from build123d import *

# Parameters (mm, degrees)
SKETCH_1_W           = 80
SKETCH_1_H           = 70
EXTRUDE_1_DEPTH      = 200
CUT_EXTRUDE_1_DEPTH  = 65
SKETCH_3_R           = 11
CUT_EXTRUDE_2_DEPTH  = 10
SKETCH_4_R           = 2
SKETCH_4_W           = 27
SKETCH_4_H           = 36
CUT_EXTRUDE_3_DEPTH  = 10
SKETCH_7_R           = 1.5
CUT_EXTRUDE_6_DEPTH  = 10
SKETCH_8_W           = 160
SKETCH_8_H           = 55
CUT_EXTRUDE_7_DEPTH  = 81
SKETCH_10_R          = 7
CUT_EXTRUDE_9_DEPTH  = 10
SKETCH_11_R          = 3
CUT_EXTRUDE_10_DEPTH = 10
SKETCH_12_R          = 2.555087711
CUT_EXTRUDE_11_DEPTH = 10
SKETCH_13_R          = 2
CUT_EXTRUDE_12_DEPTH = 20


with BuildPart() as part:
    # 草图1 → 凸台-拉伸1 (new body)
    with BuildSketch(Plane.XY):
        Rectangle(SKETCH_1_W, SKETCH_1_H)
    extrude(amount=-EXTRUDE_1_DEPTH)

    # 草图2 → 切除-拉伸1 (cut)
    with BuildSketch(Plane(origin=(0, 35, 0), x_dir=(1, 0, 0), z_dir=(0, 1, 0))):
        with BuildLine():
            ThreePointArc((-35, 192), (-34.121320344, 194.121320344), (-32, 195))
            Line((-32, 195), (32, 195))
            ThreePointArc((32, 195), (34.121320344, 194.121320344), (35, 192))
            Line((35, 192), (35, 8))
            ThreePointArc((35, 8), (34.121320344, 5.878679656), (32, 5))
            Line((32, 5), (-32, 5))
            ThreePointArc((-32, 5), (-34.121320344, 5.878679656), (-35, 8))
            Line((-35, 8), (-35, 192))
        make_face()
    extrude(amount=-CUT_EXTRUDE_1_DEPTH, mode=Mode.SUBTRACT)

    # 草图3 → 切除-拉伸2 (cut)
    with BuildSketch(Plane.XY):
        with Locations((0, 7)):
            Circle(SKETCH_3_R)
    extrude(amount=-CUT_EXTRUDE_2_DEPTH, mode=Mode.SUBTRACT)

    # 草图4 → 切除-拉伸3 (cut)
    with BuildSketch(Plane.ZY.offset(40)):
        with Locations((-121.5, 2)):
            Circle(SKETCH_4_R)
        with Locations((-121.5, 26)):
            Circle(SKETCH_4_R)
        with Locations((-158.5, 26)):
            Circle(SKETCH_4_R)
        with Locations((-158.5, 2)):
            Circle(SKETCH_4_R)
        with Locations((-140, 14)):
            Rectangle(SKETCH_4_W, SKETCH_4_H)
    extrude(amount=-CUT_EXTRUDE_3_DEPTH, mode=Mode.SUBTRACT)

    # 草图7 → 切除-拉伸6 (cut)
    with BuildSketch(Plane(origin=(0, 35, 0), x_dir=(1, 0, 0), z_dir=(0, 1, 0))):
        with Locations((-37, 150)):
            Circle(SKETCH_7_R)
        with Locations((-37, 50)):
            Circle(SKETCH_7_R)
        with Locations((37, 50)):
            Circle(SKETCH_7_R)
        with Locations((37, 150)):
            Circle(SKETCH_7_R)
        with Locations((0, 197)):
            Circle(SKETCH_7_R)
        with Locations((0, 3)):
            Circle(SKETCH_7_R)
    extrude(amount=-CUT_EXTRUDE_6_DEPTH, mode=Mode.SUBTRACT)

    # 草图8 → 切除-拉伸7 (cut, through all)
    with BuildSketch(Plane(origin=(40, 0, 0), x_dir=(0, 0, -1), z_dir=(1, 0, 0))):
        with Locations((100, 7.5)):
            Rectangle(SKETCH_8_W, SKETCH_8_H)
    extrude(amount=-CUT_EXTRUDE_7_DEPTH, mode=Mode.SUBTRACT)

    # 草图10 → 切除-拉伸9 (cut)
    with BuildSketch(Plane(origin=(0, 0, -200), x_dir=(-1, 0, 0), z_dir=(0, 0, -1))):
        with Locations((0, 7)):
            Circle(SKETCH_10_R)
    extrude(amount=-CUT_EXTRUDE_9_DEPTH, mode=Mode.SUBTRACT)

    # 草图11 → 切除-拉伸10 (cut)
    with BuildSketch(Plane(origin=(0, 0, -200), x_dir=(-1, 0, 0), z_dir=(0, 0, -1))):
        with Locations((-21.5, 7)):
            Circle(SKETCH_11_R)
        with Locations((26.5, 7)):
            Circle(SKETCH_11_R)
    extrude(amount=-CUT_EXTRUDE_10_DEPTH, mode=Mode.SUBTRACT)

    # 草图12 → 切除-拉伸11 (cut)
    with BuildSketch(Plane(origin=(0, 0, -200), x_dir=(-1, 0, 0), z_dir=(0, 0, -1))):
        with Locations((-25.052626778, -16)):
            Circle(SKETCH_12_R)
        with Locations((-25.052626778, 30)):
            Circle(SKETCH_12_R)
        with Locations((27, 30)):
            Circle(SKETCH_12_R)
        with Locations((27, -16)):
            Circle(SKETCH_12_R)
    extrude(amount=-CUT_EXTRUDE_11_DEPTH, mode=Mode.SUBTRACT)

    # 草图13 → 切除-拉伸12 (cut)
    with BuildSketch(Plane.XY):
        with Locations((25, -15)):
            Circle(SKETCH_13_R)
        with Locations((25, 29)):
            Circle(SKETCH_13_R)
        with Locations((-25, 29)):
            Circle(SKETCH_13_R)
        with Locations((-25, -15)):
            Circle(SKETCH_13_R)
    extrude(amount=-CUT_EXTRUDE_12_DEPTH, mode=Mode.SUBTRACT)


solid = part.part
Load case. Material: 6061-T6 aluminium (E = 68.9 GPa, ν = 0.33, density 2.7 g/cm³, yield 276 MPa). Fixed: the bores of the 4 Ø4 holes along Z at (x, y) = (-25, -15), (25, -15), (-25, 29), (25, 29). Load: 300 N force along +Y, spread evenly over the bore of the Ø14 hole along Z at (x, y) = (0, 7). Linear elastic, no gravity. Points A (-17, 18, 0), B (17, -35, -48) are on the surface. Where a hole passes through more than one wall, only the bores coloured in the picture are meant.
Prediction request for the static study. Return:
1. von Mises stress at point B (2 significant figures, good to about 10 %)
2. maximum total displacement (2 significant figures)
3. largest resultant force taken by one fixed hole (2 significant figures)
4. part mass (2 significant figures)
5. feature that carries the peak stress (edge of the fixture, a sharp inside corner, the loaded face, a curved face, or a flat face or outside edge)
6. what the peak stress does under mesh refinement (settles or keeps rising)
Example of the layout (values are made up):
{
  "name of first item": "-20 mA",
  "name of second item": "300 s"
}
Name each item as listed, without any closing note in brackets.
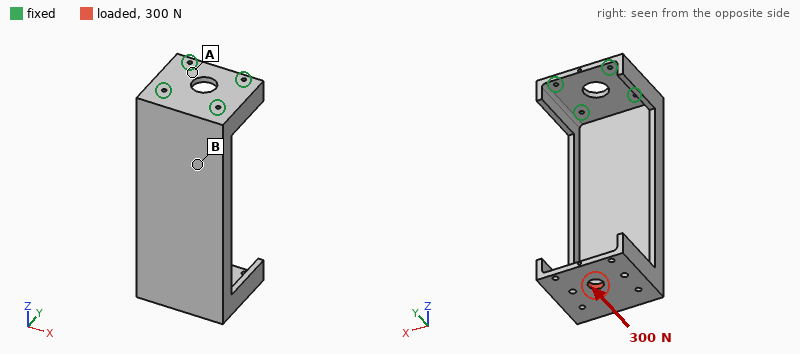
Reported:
{
  "von Mises stress at point B": "27 MPa",
  "maximum total displacement": "2.3 mm",
  "largest resultant force taken by one fixed hole": "740 N",
  "part mass": "440 g",
  "feature that carries the peak stress": "edge of the fixture",
  "what the peak stress does under mesh refinement": "keeps rising"
}
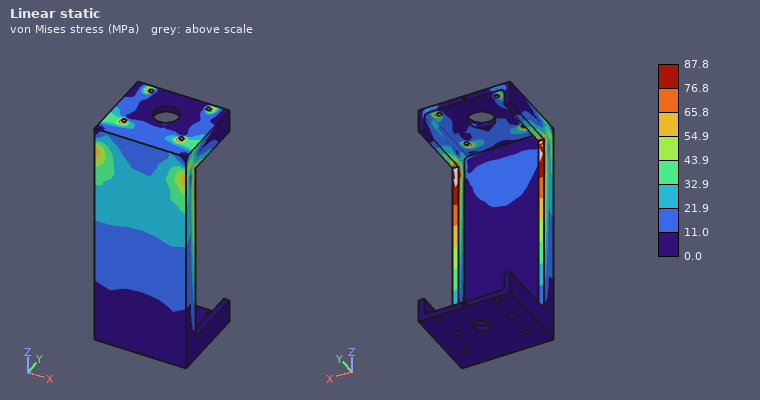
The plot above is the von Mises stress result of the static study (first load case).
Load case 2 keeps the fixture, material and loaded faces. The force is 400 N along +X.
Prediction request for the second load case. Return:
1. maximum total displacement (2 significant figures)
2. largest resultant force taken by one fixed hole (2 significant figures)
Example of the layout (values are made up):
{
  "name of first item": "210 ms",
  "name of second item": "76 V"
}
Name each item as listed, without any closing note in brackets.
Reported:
{
  "maximum total displacement": "1.8 mm",
  "largest resultant force taken by one fixed hole": "1.9 kN"
}
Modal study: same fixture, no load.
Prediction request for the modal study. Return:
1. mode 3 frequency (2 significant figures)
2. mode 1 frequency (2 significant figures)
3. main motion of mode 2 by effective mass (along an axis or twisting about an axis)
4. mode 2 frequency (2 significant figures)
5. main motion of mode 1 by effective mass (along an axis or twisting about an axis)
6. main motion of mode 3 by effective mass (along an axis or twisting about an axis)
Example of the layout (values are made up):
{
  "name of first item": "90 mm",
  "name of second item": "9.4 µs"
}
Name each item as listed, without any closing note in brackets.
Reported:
{
  "mode 3 frequency": "630 Hz",
  "mode 1 frequency": "150 Hz",
  "main motion of mode 2 by effective mass": "along X",
  "mode 2 frequency": "260 Hz",
  "main motion of mode 1 by effective mass": "along Y",
  "main motion of mode 3 by effective mass": "along X"
}
